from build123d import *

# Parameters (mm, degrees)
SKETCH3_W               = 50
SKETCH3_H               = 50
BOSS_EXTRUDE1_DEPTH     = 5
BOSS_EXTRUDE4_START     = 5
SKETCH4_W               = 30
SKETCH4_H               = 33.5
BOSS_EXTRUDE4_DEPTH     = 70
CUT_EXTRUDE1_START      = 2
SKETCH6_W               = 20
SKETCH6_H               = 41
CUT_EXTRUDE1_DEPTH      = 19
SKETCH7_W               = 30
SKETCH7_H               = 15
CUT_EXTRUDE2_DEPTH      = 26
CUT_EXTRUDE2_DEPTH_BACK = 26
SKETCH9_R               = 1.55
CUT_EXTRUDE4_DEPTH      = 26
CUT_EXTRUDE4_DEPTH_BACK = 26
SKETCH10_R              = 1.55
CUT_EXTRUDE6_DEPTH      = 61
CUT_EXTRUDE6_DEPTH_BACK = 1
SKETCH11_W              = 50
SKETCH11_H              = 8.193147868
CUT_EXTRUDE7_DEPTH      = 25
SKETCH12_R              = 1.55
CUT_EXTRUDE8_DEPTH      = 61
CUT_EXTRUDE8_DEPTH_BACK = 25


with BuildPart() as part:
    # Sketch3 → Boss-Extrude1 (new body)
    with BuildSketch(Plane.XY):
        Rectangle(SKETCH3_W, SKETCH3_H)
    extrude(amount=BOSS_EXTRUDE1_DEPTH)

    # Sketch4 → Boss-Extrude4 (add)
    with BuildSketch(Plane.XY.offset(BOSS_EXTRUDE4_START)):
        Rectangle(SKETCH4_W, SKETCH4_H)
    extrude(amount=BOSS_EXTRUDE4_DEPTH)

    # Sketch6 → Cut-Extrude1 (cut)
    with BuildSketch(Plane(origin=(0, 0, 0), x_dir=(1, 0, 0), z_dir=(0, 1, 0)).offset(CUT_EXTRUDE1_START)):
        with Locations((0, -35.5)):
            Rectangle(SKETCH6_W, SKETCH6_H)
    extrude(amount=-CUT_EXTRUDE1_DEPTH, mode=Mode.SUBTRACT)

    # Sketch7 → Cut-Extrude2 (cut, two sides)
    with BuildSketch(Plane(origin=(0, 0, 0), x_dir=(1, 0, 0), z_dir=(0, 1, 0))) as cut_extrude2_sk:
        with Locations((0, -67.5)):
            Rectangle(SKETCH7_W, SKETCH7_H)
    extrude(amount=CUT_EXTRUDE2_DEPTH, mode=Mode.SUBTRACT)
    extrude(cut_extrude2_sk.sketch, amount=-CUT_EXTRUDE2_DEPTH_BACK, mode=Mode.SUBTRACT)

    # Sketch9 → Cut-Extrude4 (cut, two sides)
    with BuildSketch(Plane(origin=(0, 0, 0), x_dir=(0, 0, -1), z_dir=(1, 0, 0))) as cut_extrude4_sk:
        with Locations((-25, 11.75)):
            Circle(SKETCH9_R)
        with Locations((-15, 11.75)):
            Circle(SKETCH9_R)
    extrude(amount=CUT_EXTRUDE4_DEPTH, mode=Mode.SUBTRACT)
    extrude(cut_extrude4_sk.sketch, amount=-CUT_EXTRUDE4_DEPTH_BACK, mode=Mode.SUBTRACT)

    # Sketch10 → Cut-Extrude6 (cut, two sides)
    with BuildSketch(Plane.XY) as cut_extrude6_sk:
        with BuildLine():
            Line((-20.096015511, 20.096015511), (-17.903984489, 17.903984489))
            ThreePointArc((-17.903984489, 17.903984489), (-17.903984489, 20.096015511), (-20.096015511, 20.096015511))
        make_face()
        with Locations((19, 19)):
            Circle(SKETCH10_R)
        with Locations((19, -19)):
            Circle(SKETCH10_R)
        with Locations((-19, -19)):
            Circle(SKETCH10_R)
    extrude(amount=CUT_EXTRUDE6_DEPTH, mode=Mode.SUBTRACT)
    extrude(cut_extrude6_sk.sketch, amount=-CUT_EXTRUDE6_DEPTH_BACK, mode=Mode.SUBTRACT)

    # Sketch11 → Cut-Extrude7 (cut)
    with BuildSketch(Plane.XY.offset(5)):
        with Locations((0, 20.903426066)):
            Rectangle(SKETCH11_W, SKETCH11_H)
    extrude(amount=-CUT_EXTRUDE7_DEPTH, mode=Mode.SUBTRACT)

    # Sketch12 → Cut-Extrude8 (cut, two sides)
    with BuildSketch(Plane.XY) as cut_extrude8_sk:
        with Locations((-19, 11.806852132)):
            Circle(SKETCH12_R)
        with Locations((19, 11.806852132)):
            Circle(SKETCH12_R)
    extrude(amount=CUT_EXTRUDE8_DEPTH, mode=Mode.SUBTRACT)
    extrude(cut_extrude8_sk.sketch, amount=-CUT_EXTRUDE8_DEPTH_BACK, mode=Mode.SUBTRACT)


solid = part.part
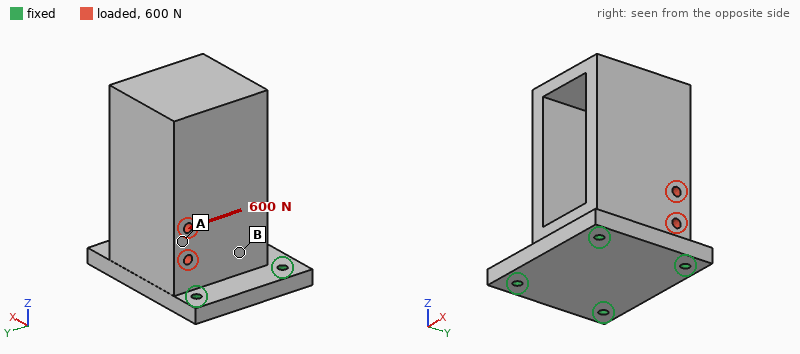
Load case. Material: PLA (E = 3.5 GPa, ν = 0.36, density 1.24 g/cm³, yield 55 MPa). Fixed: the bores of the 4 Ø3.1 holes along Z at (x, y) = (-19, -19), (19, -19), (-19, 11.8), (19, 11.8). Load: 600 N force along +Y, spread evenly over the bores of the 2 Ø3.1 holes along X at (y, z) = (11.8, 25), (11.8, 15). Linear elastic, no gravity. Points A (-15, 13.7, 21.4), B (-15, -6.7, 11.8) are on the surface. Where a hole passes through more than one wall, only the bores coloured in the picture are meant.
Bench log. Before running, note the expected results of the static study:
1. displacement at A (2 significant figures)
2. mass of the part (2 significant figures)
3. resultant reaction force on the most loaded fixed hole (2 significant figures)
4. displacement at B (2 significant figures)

0.076 mm
62 g
250 N
0.038 mm
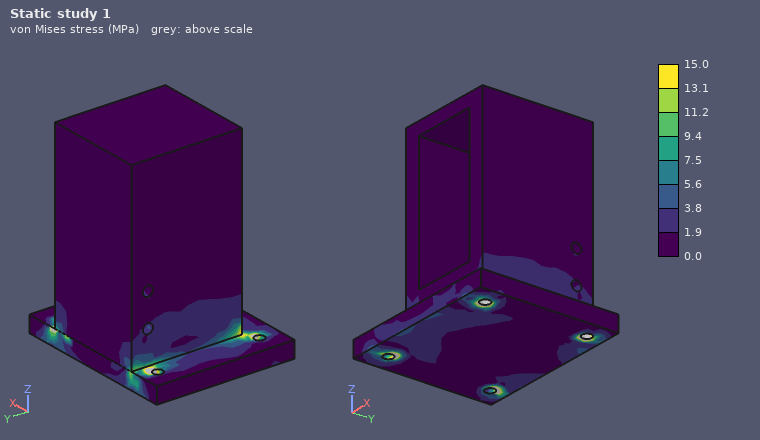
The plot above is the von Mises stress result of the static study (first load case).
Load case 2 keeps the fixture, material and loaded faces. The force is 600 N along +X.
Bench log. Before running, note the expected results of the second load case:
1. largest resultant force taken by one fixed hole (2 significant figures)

320 N
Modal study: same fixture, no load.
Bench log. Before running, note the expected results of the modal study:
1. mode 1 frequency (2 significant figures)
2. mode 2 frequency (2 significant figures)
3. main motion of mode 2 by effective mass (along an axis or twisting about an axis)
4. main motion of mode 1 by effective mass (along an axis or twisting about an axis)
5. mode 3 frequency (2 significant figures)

1200 Hz
1200 Hz
along X
along Y
2800 Hz
